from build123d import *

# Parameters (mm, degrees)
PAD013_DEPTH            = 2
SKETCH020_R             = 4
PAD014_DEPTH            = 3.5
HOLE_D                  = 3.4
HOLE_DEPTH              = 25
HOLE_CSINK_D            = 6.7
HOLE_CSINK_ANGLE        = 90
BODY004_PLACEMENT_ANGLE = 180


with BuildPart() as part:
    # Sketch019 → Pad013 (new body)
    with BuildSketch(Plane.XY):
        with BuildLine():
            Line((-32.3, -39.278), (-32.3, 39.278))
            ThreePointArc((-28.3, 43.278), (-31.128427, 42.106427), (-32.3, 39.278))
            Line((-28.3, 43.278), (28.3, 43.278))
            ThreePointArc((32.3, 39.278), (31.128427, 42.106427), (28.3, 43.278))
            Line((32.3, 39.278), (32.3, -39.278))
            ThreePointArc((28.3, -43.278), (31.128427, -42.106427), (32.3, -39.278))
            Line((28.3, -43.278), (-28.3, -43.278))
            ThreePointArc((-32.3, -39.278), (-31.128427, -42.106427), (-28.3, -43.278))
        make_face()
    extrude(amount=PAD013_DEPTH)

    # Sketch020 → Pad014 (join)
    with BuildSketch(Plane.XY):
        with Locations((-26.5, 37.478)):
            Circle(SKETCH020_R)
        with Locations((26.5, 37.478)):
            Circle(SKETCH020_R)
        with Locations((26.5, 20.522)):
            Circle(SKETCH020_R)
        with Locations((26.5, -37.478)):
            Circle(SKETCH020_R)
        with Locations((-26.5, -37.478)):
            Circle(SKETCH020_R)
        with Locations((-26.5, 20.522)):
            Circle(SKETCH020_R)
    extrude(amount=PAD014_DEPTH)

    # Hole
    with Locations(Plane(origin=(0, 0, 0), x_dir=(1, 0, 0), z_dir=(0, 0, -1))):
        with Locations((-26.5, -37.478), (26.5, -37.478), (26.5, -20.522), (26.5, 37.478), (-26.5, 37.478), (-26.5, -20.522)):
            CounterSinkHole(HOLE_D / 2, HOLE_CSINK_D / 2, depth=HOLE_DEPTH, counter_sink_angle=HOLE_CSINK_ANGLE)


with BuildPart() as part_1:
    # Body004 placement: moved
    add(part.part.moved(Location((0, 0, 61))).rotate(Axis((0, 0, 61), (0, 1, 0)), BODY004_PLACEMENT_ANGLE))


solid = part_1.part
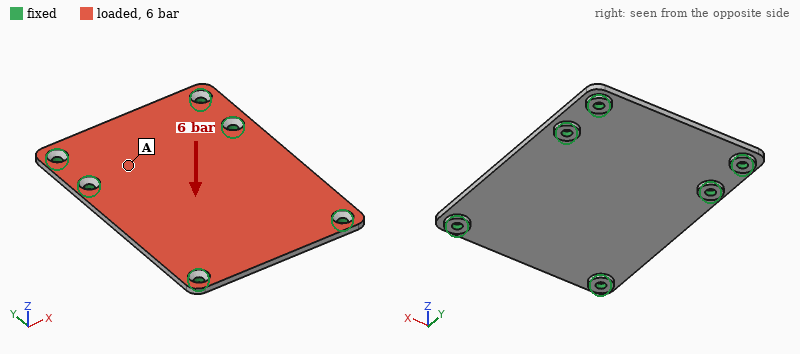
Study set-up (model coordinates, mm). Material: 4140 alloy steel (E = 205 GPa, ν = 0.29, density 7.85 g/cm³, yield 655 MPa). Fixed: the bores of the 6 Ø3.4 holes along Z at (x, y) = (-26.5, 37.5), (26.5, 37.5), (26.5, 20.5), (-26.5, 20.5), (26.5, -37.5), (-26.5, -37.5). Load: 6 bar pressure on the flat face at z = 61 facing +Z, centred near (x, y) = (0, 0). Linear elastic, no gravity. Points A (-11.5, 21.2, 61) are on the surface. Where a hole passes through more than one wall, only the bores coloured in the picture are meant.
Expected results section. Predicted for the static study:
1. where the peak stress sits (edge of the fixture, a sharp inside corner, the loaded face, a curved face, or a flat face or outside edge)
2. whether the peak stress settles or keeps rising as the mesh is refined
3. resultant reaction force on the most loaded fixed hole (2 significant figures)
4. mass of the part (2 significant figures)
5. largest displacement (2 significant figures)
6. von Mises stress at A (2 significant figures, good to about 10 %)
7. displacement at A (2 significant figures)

edge of the fixture
keeps rising
1.4 kN
89 g
0.24 mm
110 MPa
0.074 mm
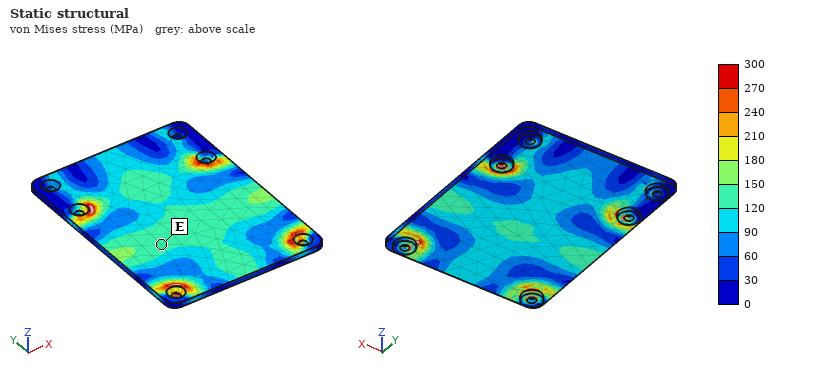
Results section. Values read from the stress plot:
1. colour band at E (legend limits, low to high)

120 to 150 MPa
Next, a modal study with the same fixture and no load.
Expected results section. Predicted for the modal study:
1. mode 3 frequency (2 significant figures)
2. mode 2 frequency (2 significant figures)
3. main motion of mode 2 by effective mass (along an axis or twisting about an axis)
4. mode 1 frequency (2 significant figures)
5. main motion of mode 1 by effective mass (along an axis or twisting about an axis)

4200 Hz
3800 Hz
twisting about Y
2400 Hz
along Z
